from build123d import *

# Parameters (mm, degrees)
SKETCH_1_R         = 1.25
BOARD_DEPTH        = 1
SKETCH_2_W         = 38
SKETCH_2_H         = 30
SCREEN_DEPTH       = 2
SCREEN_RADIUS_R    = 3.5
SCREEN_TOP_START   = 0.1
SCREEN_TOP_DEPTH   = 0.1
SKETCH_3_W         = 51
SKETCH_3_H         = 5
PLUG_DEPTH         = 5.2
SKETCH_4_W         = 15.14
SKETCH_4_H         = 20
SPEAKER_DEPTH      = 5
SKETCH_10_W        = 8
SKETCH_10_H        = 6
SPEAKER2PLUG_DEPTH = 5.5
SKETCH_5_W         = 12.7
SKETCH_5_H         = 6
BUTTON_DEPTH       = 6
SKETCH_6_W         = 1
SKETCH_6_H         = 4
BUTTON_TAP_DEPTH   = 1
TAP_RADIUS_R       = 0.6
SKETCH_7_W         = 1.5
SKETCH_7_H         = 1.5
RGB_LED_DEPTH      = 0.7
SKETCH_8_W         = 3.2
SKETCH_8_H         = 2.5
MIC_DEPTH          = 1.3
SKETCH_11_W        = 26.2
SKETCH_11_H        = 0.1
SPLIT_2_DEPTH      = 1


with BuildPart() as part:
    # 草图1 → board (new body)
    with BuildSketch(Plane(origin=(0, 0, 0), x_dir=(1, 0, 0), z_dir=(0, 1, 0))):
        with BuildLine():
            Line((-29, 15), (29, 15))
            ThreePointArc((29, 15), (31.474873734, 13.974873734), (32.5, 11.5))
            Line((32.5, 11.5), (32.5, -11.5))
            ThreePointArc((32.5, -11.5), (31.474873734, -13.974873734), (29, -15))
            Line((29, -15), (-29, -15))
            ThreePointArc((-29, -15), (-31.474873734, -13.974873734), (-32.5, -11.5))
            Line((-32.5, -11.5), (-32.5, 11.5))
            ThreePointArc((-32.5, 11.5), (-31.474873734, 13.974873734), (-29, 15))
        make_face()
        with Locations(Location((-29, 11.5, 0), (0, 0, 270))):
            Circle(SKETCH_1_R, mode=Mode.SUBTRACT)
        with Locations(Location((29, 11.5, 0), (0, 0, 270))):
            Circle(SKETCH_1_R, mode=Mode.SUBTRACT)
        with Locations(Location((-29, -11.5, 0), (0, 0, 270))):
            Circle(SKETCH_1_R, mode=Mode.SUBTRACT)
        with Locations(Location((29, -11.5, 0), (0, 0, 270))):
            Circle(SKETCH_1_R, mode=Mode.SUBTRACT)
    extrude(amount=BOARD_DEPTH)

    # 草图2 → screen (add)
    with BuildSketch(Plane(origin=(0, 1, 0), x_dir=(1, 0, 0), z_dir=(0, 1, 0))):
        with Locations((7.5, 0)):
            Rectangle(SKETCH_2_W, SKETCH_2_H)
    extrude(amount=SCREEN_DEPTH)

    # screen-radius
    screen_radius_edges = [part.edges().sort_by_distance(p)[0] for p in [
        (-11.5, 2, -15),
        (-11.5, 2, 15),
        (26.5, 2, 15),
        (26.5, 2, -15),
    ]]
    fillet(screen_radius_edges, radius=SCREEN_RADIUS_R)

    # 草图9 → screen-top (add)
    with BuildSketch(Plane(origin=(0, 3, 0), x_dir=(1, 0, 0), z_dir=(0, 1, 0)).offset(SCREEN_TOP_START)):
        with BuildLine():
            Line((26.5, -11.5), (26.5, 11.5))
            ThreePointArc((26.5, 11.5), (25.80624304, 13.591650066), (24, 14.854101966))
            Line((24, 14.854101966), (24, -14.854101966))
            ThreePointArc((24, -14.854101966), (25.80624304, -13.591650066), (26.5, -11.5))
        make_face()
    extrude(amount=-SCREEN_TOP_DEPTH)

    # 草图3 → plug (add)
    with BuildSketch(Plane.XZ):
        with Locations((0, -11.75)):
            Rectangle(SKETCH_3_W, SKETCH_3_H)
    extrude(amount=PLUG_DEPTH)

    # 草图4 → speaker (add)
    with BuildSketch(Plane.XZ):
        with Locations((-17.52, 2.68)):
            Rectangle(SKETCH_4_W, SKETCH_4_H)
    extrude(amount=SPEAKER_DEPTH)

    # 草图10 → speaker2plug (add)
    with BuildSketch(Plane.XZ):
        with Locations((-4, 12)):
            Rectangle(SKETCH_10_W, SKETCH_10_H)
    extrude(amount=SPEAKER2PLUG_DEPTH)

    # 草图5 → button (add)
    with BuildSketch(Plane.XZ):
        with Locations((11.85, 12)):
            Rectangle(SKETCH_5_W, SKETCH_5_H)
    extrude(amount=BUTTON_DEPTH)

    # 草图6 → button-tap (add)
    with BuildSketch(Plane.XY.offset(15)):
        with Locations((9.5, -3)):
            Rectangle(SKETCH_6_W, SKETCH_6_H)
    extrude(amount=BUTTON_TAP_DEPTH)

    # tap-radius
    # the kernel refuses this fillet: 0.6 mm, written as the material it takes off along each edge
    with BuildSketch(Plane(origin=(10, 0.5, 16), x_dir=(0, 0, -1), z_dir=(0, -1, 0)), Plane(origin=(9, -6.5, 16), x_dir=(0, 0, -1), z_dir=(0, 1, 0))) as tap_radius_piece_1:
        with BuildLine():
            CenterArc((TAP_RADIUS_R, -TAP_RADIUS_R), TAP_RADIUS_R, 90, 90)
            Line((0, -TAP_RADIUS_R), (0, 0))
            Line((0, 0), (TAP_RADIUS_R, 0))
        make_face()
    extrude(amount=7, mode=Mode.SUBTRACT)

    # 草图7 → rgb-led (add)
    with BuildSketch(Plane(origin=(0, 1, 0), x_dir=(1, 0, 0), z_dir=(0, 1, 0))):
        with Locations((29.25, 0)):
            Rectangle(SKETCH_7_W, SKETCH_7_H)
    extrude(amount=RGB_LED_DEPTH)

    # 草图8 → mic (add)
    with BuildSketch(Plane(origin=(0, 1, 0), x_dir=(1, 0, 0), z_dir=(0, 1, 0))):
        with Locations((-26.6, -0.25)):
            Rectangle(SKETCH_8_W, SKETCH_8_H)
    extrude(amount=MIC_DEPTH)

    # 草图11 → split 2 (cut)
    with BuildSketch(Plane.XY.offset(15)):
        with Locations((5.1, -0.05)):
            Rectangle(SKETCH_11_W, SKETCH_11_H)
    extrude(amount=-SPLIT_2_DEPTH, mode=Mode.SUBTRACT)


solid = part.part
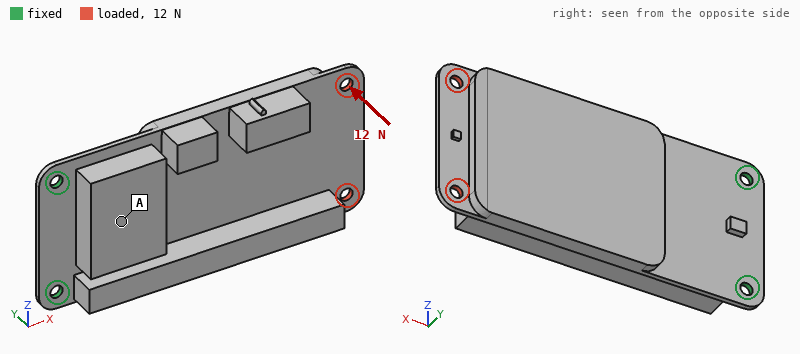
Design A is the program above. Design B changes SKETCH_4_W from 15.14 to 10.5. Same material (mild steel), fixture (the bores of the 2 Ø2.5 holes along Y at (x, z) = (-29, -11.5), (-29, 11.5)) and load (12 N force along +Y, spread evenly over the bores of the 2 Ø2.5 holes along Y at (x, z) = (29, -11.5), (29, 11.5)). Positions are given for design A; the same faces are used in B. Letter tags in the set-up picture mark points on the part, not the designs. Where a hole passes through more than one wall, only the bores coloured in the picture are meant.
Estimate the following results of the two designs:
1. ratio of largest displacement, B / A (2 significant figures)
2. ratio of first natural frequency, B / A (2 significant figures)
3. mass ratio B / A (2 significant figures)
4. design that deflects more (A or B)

1.2
0.91
0.94
B
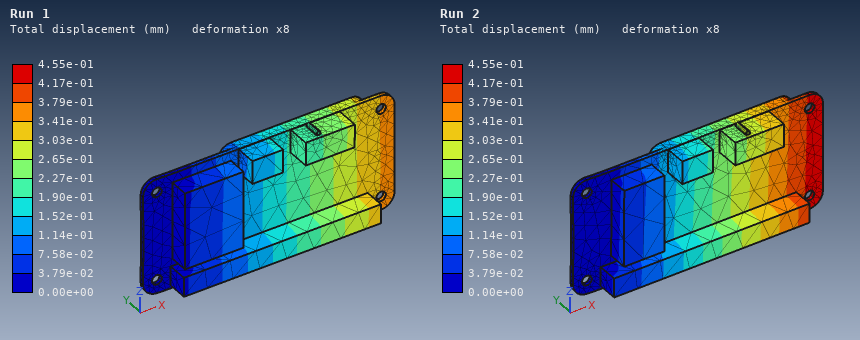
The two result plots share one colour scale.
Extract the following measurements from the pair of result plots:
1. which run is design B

Run 2
